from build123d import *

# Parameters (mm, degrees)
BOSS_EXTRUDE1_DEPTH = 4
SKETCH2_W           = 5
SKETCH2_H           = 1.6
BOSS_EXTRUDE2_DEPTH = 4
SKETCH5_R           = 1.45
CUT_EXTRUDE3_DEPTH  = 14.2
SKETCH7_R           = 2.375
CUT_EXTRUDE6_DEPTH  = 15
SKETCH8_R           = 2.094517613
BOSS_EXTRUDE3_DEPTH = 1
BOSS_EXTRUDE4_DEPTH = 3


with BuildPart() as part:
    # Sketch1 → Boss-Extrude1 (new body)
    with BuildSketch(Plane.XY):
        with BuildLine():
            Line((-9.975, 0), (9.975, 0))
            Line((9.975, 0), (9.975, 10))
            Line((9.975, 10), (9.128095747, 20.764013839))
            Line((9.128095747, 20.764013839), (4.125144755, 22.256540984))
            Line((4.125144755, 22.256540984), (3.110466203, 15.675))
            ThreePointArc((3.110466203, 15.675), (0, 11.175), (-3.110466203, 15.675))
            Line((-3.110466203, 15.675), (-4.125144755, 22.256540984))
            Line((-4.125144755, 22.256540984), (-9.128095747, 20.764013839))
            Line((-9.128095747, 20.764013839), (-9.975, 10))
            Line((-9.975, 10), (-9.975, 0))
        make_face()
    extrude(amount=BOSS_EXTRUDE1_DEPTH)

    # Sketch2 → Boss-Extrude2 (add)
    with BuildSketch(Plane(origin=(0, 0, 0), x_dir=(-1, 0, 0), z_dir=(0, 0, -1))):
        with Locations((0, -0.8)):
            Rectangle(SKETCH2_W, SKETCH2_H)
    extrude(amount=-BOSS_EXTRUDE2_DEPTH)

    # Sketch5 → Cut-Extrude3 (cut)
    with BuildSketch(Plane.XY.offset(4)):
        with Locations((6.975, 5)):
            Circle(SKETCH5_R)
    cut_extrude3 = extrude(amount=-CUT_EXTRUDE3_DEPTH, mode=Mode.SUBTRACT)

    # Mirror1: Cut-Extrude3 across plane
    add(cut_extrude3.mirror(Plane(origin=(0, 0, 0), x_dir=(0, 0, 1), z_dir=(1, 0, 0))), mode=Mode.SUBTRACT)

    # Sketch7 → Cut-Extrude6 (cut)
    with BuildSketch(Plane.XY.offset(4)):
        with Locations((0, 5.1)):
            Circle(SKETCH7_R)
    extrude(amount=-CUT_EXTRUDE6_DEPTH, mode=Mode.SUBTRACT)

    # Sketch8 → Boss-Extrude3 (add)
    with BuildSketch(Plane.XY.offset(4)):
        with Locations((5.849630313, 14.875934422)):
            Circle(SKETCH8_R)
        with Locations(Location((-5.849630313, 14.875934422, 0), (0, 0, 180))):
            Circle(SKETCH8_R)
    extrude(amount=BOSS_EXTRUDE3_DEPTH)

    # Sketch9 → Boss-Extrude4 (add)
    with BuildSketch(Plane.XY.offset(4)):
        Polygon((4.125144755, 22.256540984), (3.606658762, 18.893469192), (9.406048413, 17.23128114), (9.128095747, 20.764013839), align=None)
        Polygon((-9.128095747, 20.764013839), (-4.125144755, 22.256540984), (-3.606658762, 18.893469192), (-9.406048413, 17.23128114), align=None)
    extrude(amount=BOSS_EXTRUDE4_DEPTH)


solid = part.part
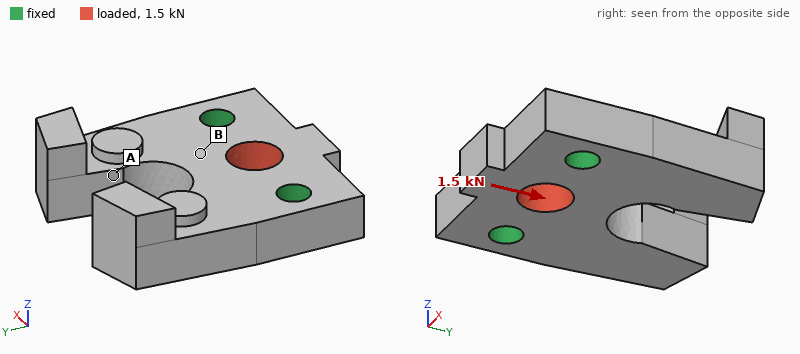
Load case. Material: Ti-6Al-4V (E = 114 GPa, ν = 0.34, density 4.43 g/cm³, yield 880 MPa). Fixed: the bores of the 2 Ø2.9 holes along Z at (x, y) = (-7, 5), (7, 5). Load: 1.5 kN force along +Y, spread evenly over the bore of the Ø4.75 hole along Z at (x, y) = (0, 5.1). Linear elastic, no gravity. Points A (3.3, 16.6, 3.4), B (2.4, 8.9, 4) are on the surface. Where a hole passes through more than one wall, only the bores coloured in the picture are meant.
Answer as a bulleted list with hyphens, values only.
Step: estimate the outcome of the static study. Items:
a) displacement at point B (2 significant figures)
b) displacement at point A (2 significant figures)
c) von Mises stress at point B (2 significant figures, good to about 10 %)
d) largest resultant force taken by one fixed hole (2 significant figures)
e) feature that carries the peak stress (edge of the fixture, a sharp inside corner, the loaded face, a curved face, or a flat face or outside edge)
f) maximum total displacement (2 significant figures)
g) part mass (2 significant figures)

- 2.2 µm
- 3.1 µm
- 32 MPa
- 750 N
- edge of the fixture
- 4.6 µm
- 6.5 g
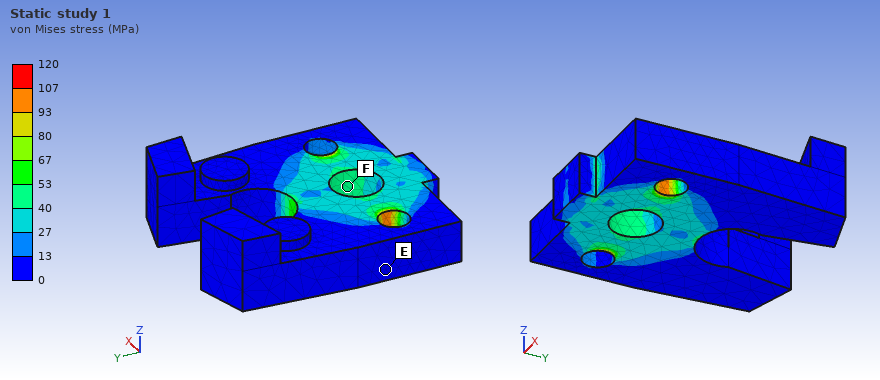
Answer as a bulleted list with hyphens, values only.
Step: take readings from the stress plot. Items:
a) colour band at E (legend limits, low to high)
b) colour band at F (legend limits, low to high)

- 0 to 13 MPa
- 40 to 53 MPa
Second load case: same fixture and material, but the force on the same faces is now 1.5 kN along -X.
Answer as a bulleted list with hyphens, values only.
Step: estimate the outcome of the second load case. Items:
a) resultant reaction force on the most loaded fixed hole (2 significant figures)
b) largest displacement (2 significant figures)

- 750 N
- 1.6 µm
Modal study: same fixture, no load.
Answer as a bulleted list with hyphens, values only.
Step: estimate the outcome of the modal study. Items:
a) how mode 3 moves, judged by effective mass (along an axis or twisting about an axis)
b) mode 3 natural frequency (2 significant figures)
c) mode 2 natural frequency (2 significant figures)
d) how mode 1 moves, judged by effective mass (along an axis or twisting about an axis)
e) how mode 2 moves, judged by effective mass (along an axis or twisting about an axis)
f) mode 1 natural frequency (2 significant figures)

- along X
- 23 kHz
- 13 kHz
- along Z
- twisting about Y
- 12 kHz
